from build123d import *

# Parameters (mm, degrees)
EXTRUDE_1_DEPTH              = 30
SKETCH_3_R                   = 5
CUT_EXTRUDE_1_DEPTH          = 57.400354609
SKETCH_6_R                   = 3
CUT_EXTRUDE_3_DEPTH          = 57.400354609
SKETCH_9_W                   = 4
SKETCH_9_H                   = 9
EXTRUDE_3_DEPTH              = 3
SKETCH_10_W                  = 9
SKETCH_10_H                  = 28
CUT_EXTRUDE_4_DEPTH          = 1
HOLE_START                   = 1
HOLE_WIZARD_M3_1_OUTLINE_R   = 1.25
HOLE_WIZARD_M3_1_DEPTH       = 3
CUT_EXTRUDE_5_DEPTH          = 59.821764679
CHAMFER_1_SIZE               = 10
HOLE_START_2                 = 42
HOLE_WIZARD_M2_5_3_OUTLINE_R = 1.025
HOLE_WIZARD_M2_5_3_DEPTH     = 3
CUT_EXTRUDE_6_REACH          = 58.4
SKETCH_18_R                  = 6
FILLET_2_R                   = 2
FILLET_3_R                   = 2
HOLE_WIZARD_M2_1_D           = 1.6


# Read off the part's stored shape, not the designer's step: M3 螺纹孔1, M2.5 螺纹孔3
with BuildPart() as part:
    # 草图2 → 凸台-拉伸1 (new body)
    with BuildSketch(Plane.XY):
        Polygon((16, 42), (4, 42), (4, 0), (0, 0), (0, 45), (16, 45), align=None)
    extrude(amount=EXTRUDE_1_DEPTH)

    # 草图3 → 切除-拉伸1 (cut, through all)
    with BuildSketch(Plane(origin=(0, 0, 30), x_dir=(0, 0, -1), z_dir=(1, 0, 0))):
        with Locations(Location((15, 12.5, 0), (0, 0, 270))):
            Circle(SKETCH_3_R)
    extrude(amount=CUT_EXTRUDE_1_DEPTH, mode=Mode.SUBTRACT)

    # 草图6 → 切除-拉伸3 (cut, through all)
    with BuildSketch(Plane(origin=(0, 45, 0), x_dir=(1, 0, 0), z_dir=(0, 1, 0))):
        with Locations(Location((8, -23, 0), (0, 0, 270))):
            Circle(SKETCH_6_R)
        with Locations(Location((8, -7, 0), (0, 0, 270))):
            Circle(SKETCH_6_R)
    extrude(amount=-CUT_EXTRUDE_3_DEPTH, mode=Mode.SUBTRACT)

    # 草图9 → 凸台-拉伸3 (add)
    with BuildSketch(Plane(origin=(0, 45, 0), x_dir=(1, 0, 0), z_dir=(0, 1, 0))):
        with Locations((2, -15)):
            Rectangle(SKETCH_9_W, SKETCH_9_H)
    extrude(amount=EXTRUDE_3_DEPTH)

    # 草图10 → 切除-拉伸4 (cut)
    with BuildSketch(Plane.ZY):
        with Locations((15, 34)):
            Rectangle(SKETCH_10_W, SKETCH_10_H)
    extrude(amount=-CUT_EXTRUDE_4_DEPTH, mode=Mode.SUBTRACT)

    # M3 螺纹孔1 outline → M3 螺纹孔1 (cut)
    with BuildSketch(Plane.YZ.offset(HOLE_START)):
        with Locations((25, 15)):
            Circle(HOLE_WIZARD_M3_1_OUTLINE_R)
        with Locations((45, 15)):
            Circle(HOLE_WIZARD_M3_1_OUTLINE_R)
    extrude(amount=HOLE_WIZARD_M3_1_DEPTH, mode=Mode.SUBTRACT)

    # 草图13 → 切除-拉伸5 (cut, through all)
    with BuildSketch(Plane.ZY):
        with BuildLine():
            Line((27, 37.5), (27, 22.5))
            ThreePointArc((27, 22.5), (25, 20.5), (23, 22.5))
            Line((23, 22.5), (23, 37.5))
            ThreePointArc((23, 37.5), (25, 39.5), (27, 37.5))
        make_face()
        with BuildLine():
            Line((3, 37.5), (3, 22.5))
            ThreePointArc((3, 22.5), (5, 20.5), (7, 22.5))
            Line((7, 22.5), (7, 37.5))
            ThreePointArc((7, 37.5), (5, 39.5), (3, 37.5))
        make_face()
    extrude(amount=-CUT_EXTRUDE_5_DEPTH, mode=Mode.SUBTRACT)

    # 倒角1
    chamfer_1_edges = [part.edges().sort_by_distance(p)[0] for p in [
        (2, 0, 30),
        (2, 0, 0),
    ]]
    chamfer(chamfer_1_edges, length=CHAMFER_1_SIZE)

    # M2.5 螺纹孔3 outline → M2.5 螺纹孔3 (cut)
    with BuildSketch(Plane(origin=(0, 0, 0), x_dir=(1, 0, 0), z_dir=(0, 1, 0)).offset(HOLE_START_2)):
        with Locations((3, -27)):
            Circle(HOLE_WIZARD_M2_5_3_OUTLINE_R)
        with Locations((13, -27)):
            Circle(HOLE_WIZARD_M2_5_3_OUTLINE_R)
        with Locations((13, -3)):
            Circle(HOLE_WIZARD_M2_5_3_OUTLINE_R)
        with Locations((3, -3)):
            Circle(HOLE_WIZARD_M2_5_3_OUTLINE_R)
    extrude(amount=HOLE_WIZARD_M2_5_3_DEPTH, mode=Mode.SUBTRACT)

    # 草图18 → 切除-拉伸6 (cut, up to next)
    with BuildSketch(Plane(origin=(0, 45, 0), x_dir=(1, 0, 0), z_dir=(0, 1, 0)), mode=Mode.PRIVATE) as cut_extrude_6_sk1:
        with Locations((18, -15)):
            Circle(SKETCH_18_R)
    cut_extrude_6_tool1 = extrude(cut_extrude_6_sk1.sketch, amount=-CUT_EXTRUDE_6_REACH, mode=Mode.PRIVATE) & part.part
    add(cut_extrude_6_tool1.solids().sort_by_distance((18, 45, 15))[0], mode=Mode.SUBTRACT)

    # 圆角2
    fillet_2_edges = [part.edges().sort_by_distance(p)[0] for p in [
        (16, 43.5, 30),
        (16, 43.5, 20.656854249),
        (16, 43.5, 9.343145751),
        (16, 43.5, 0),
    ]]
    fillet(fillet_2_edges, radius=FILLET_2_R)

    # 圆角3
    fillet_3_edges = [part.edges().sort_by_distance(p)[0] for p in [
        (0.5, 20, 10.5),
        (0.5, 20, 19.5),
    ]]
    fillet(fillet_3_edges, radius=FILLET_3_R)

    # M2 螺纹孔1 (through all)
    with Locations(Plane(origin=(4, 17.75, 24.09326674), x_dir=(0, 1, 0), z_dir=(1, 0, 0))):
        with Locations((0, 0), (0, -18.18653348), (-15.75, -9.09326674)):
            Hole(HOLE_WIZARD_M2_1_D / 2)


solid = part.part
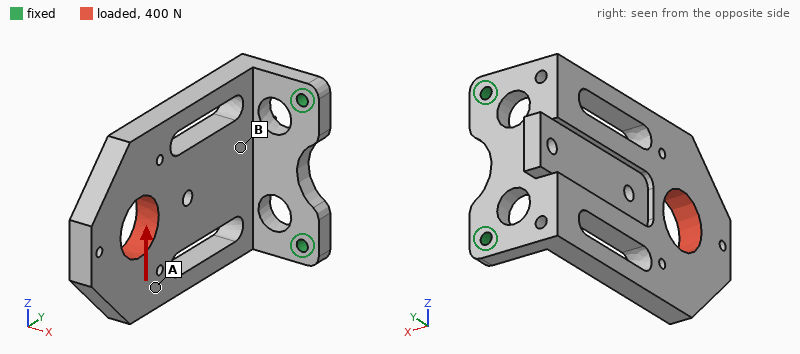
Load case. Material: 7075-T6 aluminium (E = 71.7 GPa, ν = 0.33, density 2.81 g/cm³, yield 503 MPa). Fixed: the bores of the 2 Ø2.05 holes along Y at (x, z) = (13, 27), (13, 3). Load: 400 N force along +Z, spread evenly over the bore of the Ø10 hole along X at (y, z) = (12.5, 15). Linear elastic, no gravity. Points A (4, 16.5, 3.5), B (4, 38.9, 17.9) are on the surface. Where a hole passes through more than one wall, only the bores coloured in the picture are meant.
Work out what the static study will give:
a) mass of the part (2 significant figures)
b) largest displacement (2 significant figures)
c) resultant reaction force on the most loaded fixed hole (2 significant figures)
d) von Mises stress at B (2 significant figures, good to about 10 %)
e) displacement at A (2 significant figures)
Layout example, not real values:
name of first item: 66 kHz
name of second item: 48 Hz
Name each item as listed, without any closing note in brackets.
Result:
mass of the part: 13 g
largest displacement: 0.31 mm
resultant reaction force on the most loaded fixed hole: 560 N
von Mises stress at B: 55 MPa
displacement at A: 0.22 mm
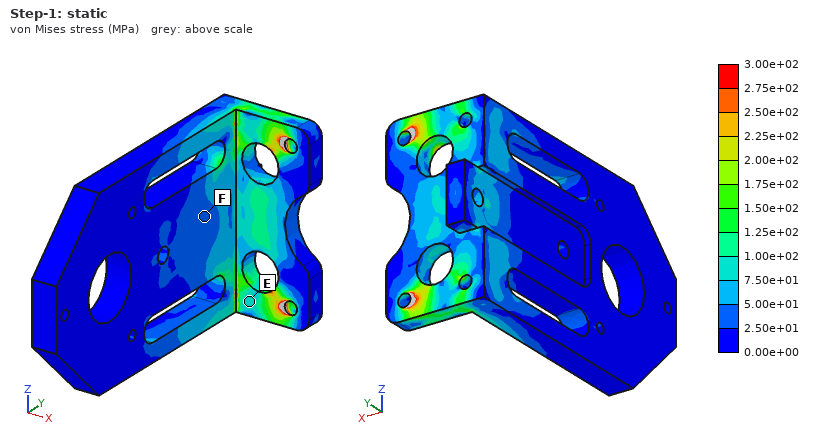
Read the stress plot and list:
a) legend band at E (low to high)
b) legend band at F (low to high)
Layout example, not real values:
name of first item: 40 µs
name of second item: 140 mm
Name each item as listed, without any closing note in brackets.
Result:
legend band at E: 7.50e+01 to 1.00e+02 MPa
legend band at F: 2.50e+01 to 5.00e+01 MPa
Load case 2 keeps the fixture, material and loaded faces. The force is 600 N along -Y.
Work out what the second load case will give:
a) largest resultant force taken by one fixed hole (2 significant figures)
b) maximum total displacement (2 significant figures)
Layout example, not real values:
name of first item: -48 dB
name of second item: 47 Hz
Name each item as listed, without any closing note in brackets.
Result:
largest resultant force taken by one fixed hole: 300 N
maximum total displacement: 0.67 mm
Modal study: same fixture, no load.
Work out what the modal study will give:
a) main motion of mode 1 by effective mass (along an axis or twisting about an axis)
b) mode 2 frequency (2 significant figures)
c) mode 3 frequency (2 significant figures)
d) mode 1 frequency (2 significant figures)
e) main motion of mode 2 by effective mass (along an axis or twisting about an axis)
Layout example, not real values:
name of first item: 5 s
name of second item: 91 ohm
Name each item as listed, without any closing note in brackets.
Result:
main motion of mode 1 by effective mass: along X
mode 2 frequency: 2500 Hz
mode 3 frequency: 4600 Hz
mode 1 frequency: 890 Hz
main motion of mode 2 by effective mass: along Z
